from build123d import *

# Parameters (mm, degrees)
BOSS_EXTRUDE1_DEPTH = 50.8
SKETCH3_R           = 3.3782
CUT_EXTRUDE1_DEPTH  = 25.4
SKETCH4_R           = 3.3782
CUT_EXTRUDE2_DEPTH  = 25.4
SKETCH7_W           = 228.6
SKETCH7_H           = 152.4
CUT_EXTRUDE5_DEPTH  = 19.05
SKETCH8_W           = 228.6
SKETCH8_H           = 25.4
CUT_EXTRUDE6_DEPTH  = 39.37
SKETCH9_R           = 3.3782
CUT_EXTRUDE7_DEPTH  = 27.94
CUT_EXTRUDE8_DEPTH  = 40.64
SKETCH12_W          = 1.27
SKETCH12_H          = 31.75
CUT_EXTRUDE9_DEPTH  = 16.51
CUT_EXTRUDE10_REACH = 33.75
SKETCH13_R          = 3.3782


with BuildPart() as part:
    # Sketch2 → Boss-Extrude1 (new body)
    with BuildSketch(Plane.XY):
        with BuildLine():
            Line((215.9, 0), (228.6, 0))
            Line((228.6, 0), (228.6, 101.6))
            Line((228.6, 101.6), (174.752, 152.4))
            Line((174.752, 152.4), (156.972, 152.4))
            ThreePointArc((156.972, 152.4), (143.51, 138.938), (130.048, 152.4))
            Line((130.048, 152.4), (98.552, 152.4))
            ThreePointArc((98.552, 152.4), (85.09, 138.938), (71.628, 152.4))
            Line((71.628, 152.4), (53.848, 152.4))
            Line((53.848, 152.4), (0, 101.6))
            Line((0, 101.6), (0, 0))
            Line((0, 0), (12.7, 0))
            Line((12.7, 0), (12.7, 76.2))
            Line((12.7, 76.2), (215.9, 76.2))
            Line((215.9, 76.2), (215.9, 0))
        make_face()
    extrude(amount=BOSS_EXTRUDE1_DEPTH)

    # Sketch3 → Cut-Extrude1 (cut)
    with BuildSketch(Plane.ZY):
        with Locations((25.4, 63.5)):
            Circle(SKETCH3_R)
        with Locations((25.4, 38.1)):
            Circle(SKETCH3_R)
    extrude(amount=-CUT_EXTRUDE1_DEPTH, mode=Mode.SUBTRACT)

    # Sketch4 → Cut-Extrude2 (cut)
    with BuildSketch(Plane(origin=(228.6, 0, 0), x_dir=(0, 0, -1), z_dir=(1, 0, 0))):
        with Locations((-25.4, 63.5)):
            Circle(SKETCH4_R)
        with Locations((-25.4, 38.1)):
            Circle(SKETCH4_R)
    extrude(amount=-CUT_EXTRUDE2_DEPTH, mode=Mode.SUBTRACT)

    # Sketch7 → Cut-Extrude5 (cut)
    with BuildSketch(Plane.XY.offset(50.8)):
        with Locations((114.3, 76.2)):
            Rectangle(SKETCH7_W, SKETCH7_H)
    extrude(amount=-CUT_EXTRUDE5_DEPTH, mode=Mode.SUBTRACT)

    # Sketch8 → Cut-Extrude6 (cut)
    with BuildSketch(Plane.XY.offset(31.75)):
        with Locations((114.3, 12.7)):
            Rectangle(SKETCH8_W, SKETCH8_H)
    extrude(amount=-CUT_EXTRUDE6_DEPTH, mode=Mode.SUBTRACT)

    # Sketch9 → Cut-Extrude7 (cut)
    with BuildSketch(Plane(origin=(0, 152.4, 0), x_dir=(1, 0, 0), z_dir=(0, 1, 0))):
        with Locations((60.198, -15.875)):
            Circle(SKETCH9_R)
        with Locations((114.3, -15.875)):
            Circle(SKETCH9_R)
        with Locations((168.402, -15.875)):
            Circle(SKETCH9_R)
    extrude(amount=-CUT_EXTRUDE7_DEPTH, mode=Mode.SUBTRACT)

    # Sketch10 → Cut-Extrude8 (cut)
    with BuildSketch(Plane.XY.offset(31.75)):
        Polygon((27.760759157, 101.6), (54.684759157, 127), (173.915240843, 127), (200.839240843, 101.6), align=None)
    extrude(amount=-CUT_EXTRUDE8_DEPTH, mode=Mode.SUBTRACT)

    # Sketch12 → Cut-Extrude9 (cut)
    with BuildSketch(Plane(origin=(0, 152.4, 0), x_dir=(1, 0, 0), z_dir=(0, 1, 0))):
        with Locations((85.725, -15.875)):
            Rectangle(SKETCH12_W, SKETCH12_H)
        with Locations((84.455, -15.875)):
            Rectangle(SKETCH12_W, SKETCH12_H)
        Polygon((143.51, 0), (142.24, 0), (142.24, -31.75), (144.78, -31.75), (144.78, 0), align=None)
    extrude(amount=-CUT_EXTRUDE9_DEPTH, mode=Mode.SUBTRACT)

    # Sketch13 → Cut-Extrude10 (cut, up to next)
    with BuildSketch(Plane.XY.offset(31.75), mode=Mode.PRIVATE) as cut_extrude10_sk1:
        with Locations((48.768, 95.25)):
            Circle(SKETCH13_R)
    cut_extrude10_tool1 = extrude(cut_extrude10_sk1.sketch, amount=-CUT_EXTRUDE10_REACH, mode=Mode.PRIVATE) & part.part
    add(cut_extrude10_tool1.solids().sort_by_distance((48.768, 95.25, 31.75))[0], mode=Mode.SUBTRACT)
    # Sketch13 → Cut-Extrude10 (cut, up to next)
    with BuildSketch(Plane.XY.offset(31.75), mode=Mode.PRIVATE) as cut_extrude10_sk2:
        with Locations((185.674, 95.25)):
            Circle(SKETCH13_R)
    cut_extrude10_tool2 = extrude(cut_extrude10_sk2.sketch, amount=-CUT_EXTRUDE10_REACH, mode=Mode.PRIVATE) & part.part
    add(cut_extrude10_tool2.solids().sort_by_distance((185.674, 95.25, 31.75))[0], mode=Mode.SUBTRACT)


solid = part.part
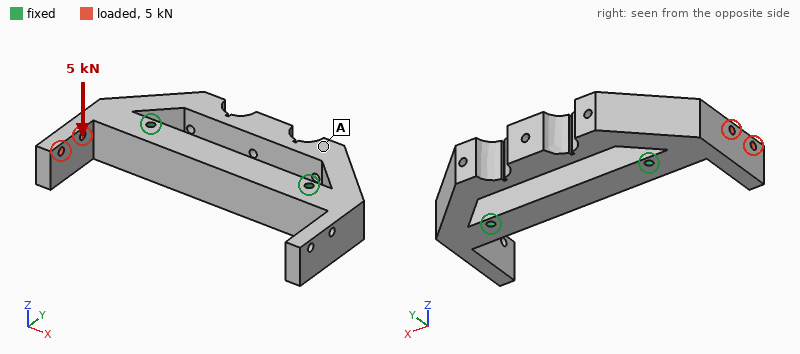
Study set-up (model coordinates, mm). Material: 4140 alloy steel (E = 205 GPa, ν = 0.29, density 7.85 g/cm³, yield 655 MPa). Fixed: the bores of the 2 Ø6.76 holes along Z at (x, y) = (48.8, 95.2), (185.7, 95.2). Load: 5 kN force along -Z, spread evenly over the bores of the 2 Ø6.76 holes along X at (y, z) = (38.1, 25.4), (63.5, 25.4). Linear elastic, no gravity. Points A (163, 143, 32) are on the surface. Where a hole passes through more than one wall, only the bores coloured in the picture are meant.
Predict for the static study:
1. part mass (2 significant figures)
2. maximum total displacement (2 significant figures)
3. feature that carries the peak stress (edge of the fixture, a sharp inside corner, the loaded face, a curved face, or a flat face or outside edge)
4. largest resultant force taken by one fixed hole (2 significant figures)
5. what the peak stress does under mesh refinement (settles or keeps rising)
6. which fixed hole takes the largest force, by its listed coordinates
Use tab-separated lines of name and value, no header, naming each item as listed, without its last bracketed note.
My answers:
part mass	2.9 kg
maximum total displacement	99 µm
feature that carries the peak stress	edge of the fixture
largest resultant force taken by one fixed hole	5.5 kN
what the peak stress does under mesh refinement	keeps rising
which fixed hole takes the largest force, by its listed coordinates	(48.8, 95.2)
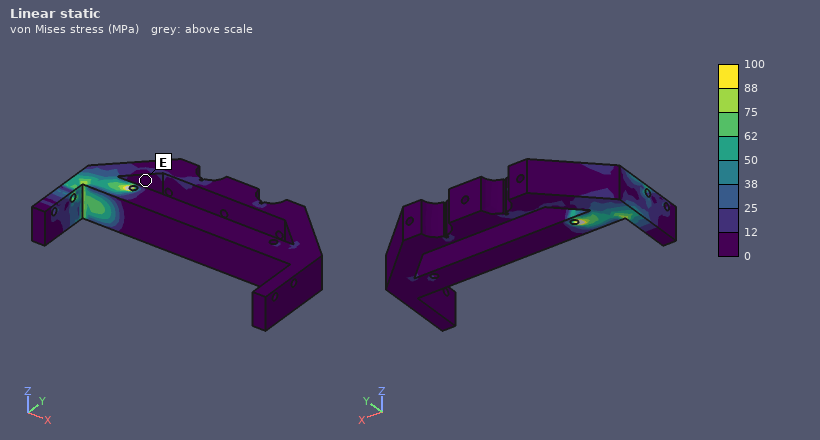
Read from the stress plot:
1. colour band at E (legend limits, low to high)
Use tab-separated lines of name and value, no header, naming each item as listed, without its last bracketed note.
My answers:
colour band at E	0 to 12 MPa
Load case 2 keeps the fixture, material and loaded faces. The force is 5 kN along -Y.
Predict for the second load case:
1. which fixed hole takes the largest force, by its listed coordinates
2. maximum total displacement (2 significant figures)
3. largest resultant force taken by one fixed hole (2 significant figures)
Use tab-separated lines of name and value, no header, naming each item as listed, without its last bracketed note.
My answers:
which fixed hole takes the largest force, by its listed coordinates	(48.8, 95.2)
maximum total displacement	54 µm
largest resultant force taken by one fixed hole	5.9 kN
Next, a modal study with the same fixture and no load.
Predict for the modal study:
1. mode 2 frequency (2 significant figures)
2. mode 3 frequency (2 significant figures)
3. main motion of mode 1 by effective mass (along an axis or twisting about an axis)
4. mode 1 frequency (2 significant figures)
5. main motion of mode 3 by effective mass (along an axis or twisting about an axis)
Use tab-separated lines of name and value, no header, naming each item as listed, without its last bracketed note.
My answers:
mode 2 frequency	2100 Hz
mode 3 frequency	2300 Hz
main motion of mode 1 by effective mass	along Z
mode 1 frequency	1800 Hz
main motion of mode 3 by effective mass	along Y
